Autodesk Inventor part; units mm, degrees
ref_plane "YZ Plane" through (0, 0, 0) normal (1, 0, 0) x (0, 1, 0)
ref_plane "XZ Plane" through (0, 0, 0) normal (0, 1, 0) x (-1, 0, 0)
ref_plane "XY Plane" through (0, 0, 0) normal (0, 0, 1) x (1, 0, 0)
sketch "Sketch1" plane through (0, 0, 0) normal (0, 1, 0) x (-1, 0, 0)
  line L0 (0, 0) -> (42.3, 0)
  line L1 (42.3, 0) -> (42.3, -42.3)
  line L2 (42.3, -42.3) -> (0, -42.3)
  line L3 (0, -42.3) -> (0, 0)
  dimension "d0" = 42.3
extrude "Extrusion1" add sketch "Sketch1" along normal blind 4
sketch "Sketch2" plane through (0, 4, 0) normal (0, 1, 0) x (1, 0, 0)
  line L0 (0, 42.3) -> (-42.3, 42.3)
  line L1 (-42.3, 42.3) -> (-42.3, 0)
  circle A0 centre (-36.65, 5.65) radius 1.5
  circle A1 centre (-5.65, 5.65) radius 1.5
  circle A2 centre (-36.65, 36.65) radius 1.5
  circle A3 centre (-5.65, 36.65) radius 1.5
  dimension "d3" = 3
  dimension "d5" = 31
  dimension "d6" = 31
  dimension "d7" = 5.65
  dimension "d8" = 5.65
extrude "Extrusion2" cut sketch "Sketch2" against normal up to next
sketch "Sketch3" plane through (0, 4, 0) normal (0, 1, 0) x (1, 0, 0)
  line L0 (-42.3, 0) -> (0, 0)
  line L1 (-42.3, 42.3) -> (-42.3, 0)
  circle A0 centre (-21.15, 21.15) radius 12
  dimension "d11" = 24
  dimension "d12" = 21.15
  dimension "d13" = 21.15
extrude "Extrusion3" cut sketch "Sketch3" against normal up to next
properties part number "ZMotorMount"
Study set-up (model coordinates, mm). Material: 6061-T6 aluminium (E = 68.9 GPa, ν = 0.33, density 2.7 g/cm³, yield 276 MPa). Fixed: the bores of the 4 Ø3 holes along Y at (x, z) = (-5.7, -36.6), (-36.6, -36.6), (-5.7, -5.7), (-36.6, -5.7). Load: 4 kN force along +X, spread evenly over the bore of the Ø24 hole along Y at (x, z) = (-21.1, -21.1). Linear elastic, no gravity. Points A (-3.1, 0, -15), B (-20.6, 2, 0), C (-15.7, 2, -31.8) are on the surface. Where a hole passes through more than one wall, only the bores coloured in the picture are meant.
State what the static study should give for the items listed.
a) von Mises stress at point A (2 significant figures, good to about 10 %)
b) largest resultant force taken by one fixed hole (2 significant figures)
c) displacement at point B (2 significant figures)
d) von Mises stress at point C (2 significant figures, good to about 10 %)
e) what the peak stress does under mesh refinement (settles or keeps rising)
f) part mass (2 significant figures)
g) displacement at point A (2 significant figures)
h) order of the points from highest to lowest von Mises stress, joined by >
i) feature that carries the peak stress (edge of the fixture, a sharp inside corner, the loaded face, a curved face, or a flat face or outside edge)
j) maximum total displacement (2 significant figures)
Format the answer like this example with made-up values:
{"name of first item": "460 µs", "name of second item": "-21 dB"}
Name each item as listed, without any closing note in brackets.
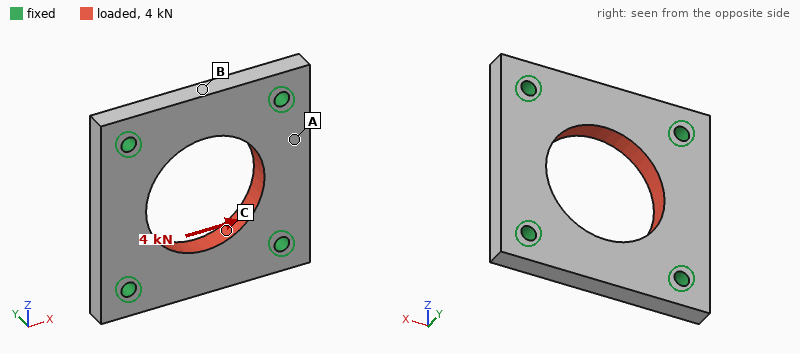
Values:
{"von Mises stress at point A": "16 MPa", "largest resultant force taken by one fixed hole": "1.0 kN", "displacement at point B": "2.5 µm", "von Mises stress at point C": "31 MPa", "what the peak stress does under mesh refinement": "keeps rising", "part mass": "14 g", "displacement at point A": "7.1 µm", "order of the points from highest to lowest von Mises stress, joined by >": "C > A > B", "feature that carries the peak stress": "edge of the fixture", "maximum total displacement": "10 µm"}
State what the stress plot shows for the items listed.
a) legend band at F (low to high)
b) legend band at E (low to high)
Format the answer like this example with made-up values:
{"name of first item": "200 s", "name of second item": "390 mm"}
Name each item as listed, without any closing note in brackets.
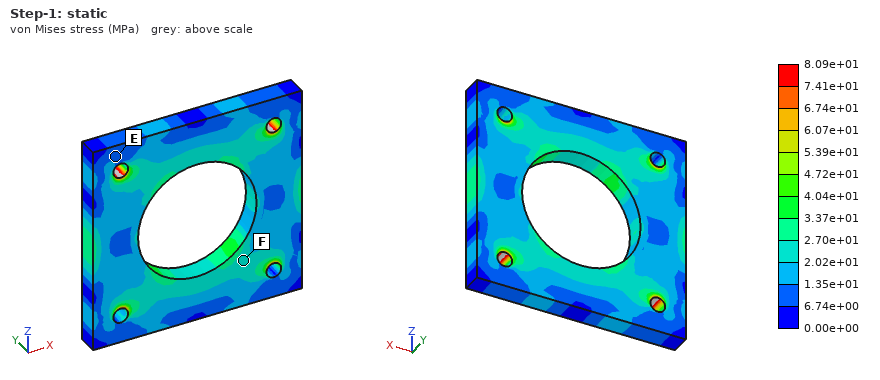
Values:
{"legend band at F": "2.02e+01 to 2.70e+01 MPa", "legend band at E": "6.74e+00 to 1.35e+01 MPa"}
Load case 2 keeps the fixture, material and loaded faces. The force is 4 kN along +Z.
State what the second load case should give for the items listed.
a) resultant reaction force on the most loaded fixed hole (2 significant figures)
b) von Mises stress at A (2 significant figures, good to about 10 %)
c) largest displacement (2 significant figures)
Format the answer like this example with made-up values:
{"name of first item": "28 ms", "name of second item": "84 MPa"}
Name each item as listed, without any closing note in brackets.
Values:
{"resultant reaction force on the most loaded fixed hole": "1.0 kN", "von Mises stress at A": "13 MPa", "largest displacement": "10 µm"}
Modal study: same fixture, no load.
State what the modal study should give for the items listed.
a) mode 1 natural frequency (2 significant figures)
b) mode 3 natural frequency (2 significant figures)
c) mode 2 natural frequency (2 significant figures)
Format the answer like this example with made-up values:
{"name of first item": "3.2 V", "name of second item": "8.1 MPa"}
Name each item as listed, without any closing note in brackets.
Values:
{"mode 1 natural frequency": "20 kHz", "mode 3 natural frequency": "21 kHz", "mode 2 natural frequency": "21 kHz"}
